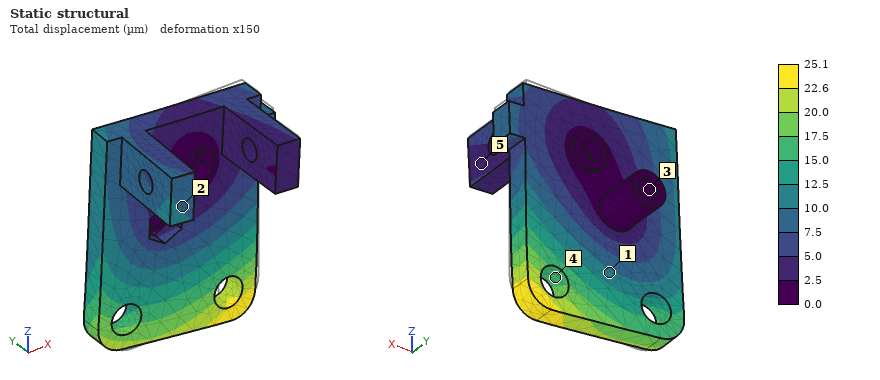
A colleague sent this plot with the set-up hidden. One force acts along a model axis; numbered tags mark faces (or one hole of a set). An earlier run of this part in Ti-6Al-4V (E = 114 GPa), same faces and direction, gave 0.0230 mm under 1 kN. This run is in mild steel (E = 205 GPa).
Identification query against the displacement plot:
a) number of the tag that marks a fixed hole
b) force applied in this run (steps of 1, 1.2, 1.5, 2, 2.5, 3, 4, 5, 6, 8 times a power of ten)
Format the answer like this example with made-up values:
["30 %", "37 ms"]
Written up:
["3", "2 kN"]
